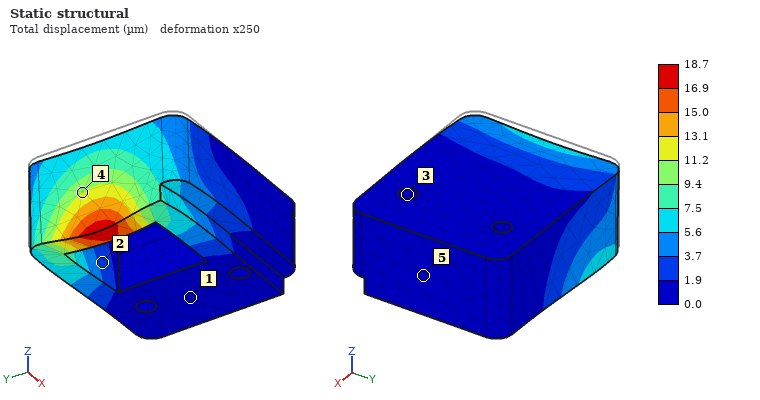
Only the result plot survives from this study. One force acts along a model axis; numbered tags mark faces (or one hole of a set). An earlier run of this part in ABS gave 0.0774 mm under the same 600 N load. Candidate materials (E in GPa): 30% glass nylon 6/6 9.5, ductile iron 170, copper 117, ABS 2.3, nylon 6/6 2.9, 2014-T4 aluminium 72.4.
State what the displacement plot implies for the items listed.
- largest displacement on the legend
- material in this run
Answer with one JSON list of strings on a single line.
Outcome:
["18.7 µm", "30% glass nylon 6/6"]
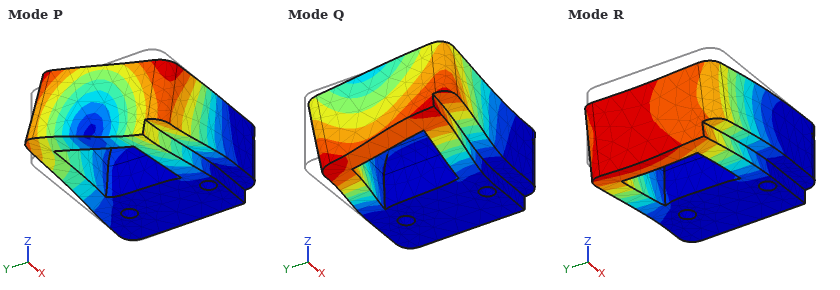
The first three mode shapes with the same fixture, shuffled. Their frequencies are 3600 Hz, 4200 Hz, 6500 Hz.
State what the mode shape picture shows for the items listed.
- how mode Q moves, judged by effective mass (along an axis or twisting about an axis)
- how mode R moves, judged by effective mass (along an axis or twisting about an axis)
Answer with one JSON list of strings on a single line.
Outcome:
["along Y", "along Z"]
